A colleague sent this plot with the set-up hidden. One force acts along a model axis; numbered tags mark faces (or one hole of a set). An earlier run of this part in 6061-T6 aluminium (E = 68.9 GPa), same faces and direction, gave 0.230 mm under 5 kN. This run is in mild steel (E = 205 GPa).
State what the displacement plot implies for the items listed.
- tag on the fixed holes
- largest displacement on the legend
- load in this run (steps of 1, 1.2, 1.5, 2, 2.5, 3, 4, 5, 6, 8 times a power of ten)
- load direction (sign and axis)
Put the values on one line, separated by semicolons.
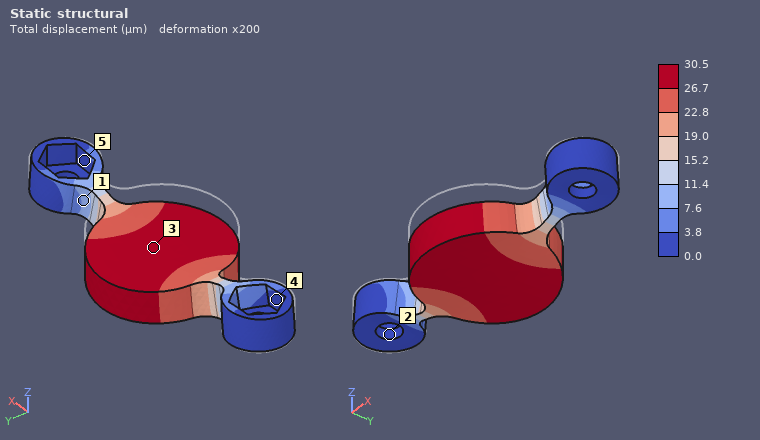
2; 30.5 µm; 2 kN; -Z
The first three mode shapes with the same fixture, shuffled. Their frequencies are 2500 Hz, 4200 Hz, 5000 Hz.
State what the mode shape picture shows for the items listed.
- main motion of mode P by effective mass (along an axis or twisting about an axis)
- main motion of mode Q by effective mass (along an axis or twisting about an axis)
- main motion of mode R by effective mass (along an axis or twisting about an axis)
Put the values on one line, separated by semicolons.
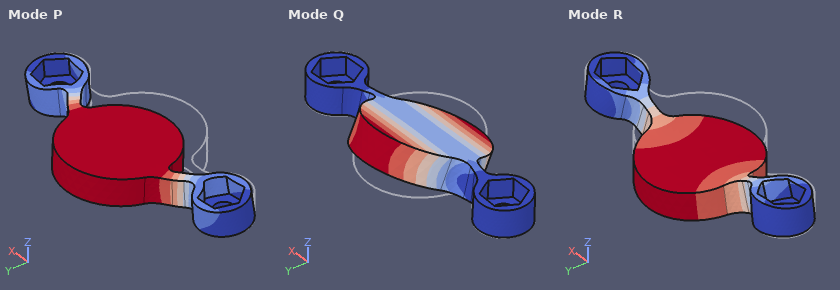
along Y; twisting about X; along Z
